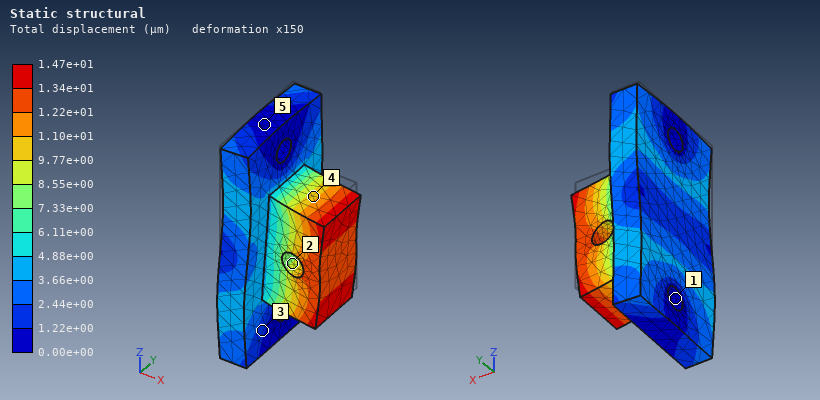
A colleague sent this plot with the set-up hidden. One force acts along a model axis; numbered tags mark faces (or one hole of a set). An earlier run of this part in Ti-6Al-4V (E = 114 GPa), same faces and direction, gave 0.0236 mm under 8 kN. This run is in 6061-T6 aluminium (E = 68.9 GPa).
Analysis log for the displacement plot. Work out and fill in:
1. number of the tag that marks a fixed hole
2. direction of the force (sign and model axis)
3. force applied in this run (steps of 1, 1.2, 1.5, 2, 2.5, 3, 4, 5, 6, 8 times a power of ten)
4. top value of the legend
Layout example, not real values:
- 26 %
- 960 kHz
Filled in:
- 1
- -Z
- 3 kN
- 1.47e+01 µm
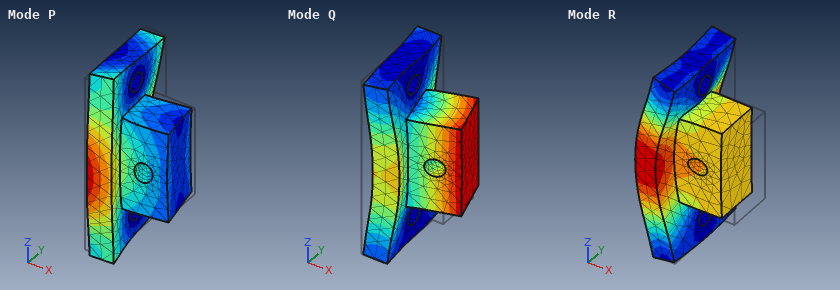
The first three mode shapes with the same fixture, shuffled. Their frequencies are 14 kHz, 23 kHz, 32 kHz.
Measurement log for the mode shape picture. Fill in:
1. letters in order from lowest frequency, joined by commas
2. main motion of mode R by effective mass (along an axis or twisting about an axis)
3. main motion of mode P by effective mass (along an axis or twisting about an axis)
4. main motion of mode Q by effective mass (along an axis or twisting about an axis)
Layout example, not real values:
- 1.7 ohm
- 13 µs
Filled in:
- Q, R, P
- along X
- along Y
- along Y
